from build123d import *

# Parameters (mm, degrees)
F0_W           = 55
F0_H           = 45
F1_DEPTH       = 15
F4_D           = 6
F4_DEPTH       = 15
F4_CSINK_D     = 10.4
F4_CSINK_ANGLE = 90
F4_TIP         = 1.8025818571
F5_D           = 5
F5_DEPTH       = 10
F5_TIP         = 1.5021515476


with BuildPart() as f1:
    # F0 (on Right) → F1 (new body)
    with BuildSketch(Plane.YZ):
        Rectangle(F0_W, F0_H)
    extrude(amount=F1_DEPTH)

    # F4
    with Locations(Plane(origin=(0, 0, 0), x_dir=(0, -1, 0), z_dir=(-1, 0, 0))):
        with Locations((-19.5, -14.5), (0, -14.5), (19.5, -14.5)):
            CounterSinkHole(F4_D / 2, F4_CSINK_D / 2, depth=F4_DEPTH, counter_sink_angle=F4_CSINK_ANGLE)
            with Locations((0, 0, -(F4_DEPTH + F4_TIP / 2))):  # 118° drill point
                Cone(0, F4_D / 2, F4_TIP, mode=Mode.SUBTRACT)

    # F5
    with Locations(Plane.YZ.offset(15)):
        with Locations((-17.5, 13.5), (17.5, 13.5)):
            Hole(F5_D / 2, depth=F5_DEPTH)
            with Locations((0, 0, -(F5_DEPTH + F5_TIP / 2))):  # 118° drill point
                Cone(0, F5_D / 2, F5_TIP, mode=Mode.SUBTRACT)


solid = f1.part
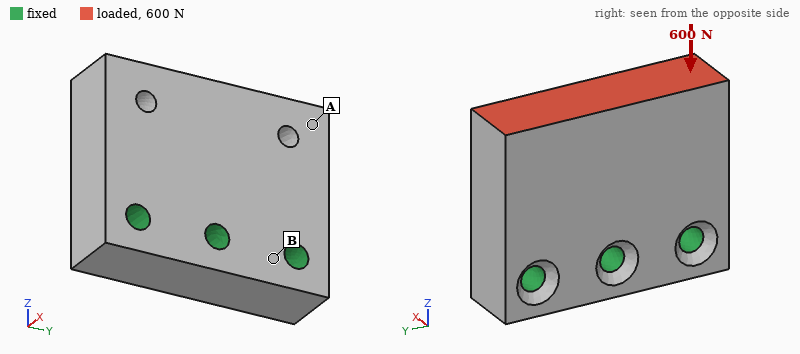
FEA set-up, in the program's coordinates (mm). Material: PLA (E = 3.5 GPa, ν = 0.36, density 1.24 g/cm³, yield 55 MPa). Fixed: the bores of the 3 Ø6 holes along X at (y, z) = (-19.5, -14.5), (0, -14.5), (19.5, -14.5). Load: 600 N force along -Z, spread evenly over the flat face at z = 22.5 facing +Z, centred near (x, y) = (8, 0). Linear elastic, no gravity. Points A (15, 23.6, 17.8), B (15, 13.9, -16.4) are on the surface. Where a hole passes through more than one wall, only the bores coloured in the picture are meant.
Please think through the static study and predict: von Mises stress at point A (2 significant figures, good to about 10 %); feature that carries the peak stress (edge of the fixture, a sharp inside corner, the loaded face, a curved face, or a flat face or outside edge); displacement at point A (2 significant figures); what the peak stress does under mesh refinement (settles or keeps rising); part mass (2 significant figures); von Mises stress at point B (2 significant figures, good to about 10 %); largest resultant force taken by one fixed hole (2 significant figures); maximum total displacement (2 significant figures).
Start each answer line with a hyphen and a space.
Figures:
- 0.91 MPa
- edge of the fixture
- 7.6 µm
- keeps rising
- 44 g
- 0.38 MPa
- 210 N
- 9.0 µm
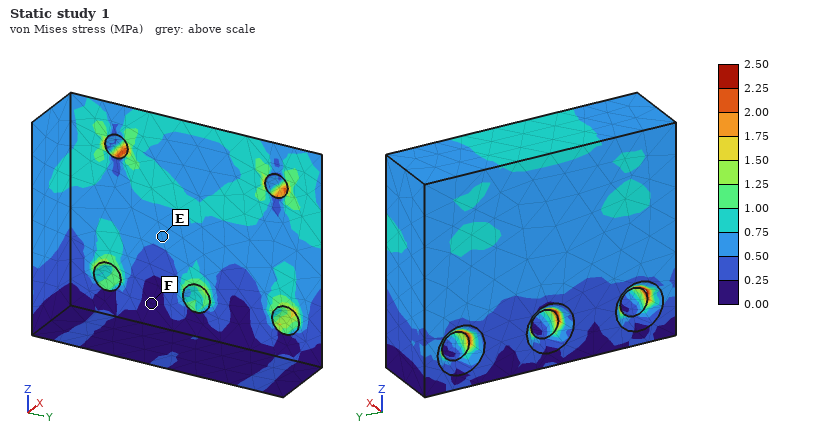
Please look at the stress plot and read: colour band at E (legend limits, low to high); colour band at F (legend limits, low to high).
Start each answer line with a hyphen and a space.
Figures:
- 0.50 to 0.75 MPa
- 0.00 to 0.25 MPa
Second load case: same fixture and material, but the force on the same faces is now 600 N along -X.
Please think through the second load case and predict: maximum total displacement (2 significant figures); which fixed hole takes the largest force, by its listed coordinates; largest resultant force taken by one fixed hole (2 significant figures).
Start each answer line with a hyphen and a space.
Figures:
- 0.24 mm
- (0, -14.5)
- 280 N
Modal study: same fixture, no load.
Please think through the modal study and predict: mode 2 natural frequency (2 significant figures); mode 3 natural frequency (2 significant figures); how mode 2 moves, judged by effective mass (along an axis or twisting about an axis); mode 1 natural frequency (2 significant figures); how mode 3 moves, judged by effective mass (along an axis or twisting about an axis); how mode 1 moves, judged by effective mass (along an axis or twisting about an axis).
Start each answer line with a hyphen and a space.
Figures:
- 4200 Hz
- 5400 Hz
- twisting about Z
- 2600 Hz
- along Y
- along X
